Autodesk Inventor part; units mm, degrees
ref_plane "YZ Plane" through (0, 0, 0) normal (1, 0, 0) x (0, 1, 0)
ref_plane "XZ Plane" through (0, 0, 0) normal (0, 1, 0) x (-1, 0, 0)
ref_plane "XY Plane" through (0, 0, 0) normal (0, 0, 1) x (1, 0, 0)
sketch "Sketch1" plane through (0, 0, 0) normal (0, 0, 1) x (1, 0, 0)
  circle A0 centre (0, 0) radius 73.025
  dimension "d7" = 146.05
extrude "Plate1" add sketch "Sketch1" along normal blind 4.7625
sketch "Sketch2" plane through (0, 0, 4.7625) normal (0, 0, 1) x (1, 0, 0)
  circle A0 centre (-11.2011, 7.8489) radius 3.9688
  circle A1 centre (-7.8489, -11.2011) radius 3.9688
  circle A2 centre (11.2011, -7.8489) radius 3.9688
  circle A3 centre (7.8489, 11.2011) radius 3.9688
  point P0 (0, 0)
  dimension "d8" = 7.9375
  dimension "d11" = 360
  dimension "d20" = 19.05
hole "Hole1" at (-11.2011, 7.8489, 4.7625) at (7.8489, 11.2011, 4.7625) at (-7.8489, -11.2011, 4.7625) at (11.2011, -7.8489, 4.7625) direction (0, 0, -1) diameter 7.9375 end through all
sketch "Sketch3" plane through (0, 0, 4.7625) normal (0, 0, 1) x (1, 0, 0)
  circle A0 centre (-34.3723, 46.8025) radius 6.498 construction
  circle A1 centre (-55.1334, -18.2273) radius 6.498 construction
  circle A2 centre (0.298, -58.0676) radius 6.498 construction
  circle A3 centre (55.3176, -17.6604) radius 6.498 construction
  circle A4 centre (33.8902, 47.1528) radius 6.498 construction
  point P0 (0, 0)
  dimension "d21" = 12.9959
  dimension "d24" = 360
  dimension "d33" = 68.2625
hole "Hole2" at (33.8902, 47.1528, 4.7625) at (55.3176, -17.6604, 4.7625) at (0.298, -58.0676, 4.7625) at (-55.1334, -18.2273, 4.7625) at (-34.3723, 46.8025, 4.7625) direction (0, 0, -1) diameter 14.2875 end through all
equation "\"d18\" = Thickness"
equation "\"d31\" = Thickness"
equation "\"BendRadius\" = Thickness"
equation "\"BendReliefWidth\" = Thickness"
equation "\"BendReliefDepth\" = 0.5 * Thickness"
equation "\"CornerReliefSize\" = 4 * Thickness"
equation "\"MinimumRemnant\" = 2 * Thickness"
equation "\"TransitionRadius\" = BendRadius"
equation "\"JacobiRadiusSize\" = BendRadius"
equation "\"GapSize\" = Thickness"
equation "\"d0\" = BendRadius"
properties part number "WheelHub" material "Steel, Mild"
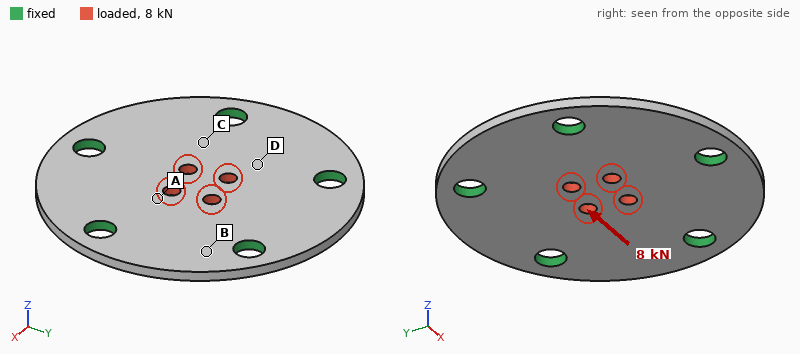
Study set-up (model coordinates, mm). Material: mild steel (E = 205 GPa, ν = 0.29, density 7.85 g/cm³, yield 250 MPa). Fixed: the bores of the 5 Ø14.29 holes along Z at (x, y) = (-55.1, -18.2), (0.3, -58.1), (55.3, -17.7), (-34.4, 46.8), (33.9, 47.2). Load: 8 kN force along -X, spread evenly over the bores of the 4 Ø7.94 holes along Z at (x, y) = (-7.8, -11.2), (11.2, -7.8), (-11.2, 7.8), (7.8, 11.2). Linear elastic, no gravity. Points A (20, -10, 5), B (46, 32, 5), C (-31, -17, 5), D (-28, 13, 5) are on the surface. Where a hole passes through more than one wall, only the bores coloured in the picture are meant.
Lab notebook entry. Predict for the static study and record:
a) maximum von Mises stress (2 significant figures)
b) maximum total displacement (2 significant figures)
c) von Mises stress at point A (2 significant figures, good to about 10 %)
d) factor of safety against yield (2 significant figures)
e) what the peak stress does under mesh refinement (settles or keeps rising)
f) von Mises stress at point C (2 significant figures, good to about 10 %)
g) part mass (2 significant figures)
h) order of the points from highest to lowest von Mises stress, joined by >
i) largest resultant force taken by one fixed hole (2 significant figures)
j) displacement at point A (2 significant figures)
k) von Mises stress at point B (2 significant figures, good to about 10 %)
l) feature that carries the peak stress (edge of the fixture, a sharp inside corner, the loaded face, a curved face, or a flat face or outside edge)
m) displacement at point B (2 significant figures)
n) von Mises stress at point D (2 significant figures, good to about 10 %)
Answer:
45 MPa
4.3 µm
18 MPa
5.6
settles
15 MPa
590 g
A > C > D > B
2.3 kN
2.5 µm
6.2 MPa
the loaded face
0.96 µm
10 MPa
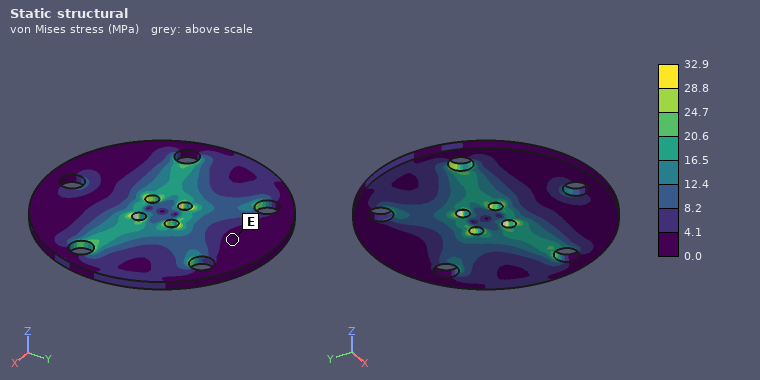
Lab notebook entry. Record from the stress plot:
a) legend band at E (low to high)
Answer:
0.0 to 4.1 MPa
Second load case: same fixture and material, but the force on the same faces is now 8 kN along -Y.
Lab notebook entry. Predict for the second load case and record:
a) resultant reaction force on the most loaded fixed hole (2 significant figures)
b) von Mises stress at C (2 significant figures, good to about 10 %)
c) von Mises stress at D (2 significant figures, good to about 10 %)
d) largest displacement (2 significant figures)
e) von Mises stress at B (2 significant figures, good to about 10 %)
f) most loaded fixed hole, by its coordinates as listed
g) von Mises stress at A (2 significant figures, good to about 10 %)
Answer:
2.3 kN
6.7 MPa
10 MPa
4.3 µm
3.1 MPa
(0.3, -58.1)
14 MPa
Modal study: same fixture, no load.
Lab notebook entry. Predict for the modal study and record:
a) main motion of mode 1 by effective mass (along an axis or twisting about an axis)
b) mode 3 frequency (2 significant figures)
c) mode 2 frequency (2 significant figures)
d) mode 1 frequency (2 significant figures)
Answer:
along Z
5400 Hz
5400 Hz
3500 Hz
